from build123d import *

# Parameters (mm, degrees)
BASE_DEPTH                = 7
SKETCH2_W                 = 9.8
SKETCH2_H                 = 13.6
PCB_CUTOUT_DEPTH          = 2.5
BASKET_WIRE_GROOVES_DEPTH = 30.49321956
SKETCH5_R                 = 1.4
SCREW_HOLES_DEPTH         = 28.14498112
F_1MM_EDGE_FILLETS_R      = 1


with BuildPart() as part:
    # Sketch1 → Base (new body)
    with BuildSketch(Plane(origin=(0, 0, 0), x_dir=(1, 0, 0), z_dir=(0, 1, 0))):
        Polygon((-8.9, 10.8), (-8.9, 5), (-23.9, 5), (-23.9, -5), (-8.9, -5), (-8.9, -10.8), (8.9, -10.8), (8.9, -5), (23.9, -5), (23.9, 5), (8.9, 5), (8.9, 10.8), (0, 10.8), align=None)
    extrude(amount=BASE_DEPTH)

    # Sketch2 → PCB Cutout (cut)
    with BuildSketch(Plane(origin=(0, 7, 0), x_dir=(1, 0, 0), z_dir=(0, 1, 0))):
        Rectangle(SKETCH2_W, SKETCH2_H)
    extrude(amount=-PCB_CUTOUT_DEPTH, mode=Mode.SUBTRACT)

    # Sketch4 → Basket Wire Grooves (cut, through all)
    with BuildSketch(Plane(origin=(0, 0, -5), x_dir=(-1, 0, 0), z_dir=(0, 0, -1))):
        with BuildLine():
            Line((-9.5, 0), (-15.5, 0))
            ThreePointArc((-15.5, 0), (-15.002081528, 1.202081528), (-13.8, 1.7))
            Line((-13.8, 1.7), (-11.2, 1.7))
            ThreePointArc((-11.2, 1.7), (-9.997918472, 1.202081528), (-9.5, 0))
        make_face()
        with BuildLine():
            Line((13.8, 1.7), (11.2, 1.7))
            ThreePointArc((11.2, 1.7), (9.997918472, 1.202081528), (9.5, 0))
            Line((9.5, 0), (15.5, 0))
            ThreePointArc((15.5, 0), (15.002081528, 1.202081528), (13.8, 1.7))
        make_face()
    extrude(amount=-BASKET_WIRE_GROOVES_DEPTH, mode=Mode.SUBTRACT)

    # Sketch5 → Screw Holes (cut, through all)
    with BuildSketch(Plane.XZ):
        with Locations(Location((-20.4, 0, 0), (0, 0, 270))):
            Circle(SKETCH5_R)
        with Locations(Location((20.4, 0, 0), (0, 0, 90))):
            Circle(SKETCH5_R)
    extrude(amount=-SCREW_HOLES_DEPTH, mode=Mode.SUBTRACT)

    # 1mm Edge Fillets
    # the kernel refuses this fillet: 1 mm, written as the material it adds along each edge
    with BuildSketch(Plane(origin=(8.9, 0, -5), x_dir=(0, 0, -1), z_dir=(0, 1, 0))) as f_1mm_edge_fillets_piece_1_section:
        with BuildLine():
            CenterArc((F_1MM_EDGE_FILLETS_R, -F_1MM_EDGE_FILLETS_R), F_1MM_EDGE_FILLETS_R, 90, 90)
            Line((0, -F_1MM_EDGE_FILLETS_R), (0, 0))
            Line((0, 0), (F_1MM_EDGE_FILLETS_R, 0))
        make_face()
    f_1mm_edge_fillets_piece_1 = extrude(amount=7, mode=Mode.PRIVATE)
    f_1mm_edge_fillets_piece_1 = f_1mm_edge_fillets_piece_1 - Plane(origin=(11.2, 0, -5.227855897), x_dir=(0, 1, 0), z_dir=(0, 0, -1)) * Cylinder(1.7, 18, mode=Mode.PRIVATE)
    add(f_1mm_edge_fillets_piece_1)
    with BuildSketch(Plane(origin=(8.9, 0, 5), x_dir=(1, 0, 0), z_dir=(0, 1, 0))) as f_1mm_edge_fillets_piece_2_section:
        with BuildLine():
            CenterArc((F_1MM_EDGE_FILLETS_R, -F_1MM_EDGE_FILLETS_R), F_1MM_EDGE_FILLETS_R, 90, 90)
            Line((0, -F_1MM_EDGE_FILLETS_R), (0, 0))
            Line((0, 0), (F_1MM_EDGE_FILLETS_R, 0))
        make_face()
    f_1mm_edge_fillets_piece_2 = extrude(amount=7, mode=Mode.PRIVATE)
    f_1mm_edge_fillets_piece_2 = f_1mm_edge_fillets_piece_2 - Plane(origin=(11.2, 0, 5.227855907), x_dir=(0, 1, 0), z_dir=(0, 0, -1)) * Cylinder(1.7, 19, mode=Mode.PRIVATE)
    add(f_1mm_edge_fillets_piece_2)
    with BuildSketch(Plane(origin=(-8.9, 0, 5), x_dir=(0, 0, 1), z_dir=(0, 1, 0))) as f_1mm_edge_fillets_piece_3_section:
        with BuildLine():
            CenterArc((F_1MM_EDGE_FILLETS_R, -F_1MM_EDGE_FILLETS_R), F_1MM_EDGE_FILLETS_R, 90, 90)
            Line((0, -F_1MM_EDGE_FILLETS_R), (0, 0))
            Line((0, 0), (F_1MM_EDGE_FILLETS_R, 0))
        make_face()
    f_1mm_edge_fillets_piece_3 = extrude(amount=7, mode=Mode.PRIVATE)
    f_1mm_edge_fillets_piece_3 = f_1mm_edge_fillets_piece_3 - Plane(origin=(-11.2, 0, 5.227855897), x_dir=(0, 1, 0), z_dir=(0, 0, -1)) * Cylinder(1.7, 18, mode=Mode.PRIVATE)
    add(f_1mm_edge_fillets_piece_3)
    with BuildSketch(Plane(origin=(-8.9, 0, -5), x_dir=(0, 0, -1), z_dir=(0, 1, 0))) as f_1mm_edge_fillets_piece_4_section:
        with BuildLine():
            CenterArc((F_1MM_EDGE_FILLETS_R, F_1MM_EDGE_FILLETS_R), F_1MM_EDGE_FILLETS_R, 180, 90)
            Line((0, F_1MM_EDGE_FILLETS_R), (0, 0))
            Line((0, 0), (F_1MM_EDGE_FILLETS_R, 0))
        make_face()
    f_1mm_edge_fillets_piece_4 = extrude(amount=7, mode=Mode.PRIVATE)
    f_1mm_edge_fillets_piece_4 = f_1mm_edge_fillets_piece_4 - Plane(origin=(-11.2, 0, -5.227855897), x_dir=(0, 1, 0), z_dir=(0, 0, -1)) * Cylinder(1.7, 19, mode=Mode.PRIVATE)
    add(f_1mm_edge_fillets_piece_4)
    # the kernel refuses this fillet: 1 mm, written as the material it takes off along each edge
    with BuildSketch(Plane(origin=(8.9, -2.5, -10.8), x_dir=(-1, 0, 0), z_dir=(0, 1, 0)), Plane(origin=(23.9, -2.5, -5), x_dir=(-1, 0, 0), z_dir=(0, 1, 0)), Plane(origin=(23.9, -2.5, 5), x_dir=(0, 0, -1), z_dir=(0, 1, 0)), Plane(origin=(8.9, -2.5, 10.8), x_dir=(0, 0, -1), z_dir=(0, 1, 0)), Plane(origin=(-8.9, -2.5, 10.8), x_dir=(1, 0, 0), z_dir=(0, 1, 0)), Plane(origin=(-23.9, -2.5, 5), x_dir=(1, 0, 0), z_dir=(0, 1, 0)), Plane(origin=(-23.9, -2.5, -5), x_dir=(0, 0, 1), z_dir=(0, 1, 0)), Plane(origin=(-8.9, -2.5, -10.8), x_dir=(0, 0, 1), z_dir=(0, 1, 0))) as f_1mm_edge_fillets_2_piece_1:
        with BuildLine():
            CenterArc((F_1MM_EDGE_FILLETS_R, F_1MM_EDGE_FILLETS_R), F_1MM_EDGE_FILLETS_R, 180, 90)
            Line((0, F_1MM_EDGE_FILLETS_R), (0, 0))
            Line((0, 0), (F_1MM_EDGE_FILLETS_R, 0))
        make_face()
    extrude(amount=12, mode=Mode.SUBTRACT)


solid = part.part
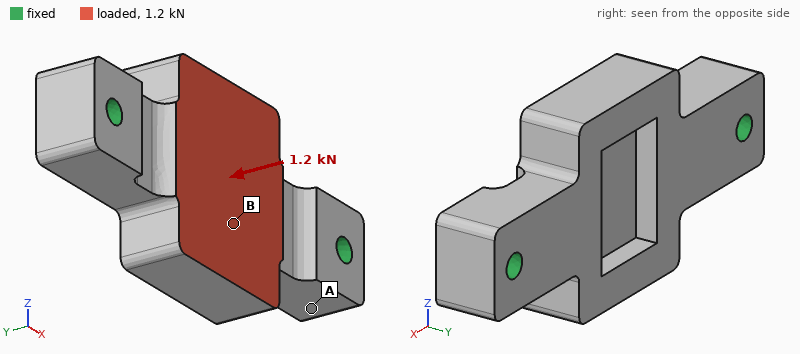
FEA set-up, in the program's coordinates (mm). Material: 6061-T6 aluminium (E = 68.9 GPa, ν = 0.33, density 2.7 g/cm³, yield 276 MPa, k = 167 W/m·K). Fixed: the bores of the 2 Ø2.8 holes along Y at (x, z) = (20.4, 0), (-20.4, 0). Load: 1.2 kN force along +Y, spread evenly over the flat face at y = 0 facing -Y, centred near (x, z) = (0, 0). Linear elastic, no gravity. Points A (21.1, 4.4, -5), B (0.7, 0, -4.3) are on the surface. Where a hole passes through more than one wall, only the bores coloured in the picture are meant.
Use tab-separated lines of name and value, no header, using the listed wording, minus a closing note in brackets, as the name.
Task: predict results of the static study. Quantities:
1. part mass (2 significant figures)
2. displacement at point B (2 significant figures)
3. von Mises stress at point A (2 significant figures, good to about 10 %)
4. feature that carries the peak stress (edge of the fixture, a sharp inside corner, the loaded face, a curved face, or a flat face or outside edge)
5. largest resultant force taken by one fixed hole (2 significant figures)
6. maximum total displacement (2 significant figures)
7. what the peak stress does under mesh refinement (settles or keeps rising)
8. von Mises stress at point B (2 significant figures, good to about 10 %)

part mass	11 g
displacement at point B	26 µm
von Mises stress at point A	15 MPa
feature that carries the peak stress	edge of the fixture
largest resultant force taken by one fixed hole	700 N
maximum total displacement	29 µm
what the peak stress does under mesh refinement	keeps rising
von Mises stress at point B	34 MPa
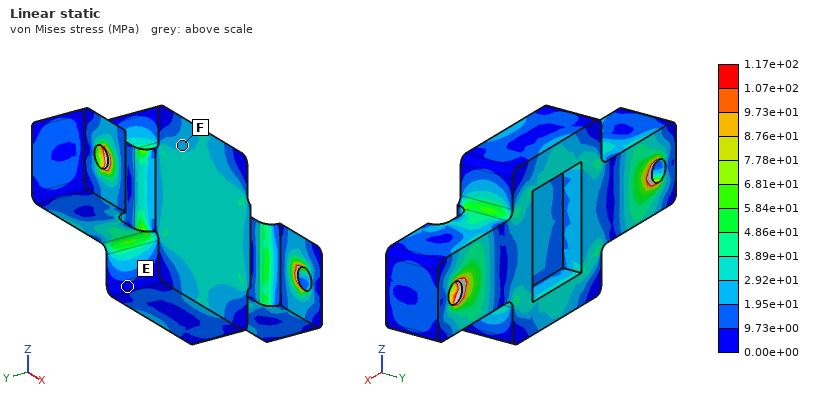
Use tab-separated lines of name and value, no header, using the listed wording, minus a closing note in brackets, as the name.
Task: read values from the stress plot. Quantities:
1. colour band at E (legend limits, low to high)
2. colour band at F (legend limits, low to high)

colour band at E	0.00e+00 to 9.73e+00 MPa
colour band at F	1.95e+01 to 2.92e+01 MPa
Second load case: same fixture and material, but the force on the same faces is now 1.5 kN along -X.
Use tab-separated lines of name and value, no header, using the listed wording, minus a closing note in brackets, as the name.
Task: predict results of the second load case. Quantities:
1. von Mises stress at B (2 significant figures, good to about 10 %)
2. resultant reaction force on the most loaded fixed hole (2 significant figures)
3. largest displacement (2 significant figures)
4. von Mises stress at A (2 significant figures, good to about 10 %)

von Mises stress at B	10.0 MPa
resultant reaction force on the most loaded fixed hole	780 N
largest displacement	7.2 µm
von Mises stress at A	4.2 MPa
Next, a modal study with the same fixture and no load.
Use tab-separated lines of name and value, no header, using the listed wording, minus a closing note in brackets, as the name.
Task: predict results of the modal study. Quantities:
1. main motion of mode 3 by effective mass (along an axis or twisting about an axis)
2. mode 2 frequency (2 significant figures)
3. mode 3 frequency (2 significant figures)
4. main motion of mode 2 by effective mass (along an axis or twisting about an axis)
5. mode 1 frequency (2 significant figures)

main motion of mode 3 by effective mass	along Z
mode 2 frequency	13 kHz
mode 3 frequency	18 kHz
main motion of mode 2 by effective mass	along Y
mode 1 frequency	12 kHz
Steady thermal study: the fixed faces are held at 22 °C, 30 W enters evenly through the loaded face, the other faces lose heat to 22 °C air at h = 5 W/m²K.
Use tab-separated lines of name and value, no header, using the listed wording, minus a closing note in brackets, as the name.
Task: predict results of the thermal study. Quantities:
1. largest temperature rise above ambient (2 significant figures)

largest temperature rise above ambient	24 K
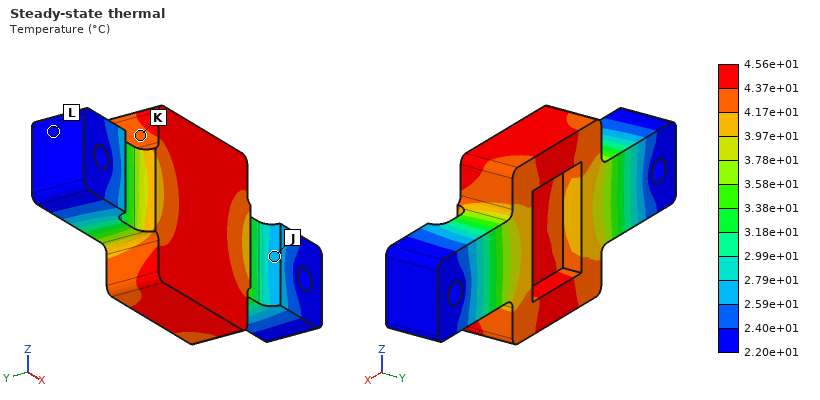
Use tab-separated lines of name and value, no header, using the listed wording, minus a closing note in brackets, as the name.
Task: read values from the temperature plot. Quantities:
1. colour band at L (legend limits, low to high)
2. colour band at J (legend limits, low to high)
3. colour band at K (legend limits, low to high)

colour band at L	2.20e+01 to 2.40e+01 °C
colour band at J	2.59e+01 to 2.79e+01 °C
colour band at K	4.17e+01 to 4.37e+01 °C
